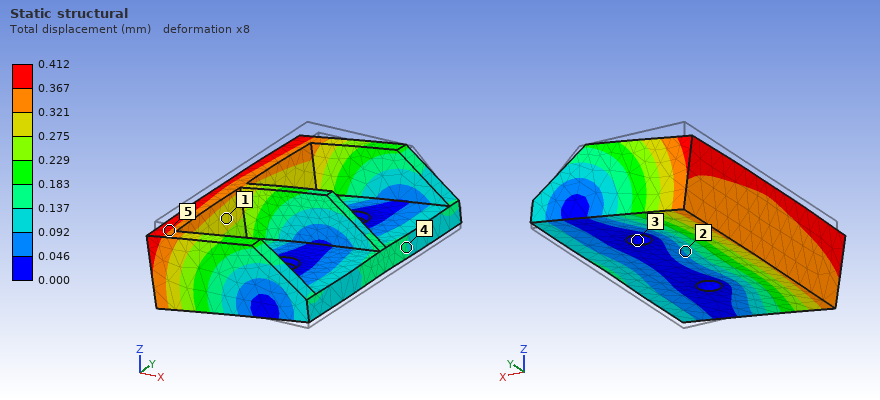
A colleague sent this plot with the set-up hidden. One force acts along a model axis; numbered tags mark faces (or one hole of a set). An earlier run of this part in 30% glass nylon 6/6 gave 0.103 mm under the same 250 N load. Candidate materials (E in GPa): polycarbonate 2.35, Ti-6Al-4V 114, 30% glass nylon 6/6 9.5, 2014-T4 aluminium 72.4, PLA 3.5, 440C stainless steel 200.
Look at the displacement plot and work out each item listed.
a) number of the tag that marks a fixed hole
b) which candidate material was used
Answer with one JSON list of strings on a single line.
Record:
["3", "polycarbonate"]
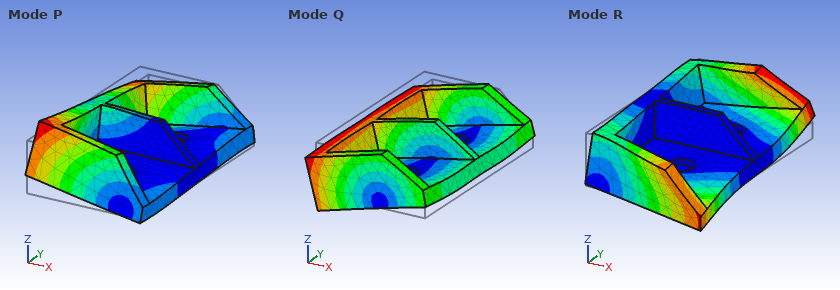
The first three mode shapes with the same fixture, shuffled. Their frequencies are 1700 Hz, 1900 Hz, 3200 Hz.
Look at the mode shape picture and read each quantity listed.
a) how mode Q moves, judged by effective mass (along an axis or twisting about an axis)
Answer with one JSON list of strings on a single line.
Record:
["along Z"]
